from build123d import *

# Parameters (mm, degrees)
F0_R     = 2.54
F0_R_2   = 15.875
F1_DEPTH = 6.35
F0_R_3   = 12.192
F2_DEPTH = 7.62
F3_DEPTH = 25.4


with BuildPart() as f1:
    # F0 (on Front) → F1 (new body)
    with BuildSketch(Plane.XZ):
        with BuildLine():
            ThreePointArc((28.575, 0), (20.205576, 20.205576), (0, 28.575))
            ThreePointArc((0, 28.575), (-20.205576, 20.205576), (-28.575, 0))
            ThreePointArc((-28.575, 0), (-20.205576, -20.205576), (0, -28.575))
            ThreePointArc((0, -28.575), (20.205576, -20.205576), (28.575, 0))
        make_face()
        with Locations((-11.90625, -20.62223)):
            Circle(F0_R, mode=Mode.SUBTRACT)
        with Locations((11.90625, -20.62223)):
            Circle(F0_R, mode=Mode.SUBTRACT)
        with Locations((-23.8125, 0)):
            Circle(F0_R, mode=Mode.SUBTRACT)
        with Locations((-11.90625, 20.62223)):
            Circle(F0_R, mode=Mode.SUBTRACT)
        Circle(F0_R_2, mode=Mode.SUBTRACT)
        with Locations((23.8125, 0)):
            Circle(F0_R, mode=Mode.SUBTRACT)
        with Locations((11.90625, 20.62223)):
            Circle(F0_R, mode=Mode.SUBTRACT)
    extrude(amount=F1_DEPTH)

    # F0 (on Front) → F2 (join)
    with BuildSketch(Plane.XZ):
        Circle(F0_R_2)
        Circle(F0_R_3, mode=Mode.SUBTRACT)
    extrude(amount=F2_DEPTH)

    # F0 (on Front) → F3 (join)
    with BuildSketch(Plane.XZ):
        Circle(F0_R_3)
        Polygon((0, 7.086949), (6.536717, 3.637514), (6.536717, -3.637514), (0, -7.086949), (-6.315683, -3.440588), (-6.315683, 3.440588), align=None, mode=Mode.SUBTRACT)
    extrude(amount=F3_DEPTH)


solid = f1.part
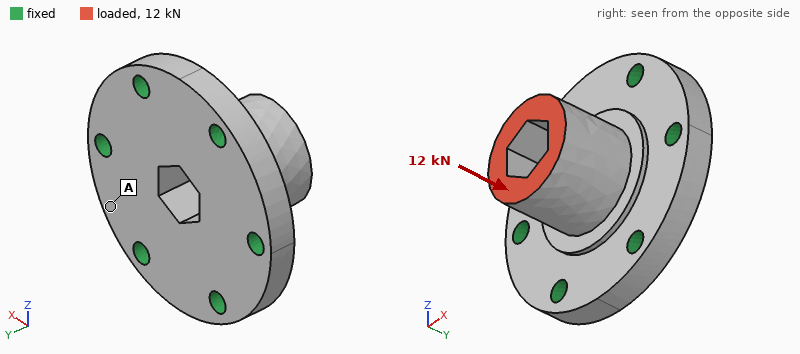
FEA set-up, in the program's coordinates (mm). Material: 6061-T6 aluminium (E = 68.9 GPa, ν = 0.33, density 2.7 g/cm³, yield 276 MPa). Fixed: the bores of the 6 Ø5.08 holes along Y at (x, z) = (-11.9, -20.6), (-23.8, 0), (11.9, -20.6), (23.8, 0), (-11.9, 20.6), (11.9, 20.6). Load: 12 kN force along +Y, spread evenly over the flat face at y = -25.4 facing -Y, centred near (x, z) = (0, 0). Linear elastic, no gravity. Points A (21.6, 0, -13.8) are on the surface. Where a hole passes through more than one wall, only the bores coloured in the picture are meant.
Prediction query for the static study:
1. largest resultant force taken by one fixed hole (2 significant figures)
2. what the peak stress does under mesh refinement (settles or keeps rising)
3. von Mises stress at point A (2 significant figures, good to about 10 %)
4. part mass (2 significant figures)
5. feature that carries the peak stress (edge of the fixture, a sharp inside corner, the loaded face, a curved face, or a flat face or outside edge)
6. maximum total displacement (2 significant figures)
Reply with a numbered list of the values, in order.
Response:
1. 2.3 kN
2. keeps rising
3. 17 MPa
4. 58 g
5. edge of the fixture
6. 37 µm
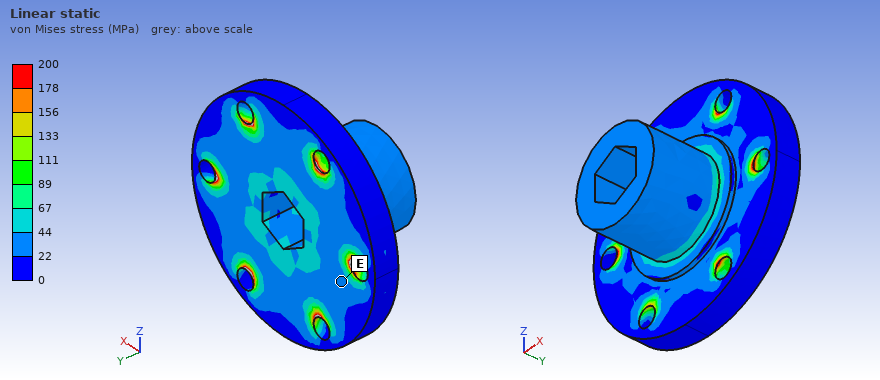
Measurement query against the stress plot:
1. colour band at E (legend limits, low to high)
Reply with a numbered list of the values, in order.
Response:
1. 22 to 44 MPa
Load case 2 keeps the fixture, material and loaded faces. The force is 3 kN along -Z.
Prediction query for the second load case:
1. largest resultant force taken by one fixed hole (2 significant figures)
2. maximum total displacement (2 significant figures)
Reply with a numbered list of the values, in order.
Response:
1. 1.2 kN
2. 40 µm
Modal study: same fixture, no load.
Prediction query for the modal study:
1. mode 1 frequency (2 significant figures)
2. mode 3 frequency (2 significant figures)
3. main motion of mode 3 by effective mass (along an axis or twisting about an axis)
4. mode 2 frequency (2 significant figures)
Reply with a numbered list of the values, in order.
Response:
1. 18 kHz
2. 19 kHz
3. along Y
4. 18 kHz
